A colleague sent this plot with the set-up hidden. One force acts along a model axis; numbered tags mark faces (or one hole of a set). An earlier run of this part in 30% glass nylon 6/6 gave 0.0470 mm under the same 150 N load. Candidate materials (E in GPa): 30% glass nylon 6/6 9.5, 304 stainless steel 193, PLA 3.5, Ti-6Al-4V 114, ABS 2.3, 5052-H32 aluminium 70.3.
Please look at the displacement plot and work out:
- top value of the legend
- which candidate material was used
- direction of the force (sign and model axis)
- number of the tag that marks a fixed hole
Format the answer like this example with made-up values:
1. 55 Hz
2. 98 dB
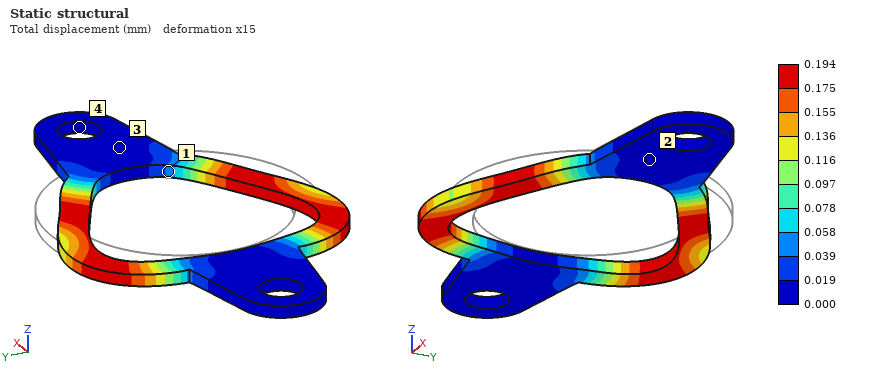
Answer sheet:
1. 0.194 mm
2. ABS
3. -X
4. 4
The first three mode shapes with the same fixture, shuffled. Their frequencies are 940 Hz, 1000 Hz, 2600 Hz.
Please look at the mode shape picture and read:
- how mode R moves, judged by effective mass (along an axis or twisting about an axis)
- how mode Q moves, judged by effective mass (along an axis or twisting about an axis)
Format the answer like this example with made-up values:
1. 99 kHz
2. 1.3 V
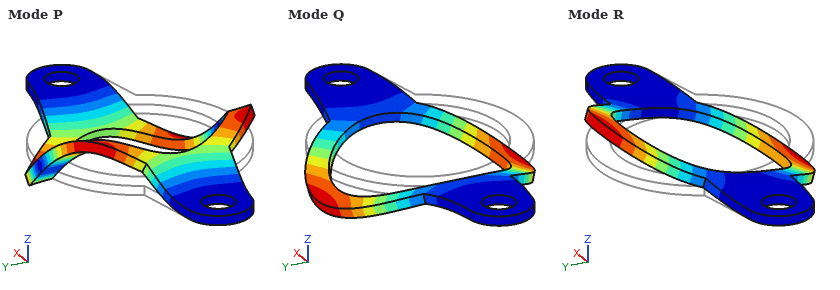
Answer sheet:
1. twisting about X
2. along Z
